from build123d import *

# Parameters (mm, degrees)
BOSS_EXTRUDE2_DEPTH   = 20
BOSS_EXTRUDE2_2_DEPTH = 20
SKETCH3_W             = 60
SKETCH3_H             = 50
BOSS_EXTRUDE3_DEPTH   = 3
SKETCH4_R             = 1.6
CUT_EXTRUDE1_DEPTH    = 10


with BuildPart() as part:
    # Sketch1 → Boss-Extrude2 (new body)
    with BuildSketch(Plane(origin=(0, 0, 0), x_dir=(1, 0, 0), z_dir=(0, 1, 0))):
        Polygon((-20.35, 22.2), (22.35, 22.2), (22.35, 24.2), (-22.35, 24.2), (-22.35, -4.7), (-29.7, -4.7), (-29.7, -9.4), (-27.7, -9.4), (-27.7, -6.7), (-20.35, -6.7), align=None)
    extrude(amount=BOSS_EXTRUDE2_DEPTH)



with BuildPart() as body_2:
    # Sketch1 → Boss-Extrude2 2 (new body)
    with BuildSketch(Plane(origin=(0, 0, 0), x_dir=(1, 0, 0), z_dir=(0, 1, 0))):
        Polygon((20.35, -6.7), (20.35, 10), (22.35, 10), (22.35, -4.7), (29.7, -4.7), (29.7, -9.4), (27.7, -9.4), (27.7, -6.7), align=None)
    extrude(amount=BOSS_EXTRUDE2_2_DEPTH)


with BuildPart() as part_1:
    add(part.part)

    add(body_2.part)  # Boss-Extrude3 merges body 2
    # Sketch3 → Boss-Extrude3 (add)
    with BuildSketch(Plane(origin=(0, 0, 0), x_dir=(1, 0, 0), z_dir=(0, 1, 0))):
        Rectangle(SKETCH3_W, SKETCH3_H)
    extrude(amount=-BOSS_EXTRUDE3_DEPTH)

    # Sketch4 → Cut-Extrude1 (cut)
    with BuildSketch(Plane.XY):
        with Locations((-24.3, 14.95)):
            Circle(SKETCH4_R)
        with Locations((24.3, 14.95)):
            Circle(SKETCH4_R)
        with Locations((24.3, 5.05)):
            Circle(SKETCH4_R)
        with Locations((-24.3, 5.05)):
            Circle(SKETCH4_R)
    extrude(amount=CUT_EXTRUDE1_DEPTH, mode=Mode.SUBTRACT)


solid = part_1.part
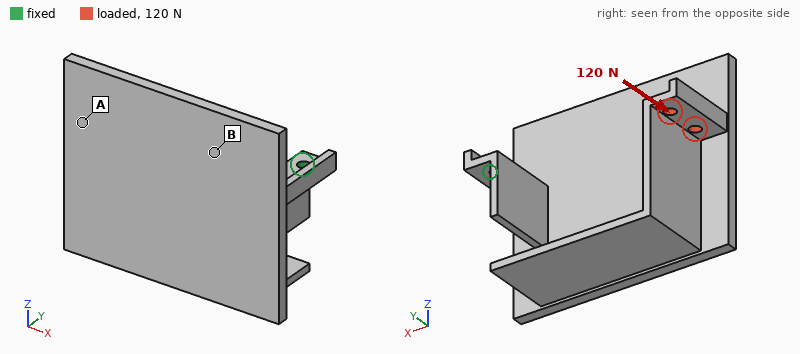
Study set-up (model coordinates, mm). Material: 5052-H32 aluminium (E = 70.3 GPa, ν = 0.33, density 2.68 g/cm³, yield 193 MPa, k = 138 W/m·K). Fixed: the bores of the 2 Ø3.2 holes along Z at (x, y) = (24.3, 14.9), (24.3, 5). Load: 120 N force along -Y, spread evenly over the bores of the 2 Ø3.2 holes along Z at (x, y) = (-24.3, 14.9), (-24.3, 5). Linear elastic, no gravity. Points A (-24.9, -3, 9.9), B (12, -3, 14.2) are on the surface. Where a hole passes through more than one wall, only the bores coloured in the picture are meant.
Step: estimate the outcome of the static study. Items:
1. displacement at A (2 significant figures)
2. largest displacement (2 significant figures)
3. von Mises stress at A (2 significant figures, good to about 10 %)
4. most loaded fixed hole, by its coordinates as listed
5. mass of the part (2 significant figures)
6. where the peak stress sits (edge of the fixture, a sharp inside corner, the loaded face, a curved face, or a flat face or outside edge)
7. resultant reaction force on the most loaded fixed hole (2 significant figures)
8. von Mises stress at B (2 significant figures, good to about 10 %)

0.74 mm
0.91 mm
17 MPa
(24.3, 5)
36 g
edge of the fixture
360 N
54 MPa
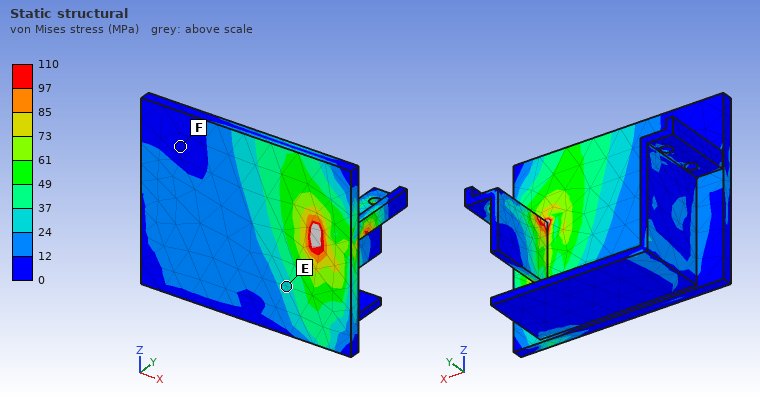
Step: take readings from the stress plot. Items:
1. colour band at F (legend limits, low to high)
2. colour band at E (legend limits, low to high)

0 to 12 MPa
24 to 37 MPa
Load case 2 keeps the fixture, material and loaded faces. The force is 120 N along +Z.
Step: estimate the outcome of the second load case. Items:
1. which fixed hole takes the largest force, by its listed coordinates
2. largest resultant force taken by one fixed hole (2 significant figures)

(24.3, 5)
110 N
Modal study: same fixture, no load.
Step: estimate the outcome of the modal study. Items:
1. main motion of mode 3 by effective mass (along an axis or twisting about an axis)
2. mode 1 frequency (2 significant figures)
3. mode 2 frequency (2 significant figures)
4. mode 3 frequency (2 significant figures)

twisting about X
540 Hz
550 Hz
1300 Hz
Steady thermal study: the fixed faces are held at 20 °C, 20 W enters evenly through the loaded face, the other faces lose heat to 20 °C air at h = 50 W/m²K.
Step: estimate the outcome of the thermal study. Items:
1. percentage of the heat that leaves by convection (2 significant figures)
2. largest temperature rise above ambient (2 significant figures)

63 %
69 K
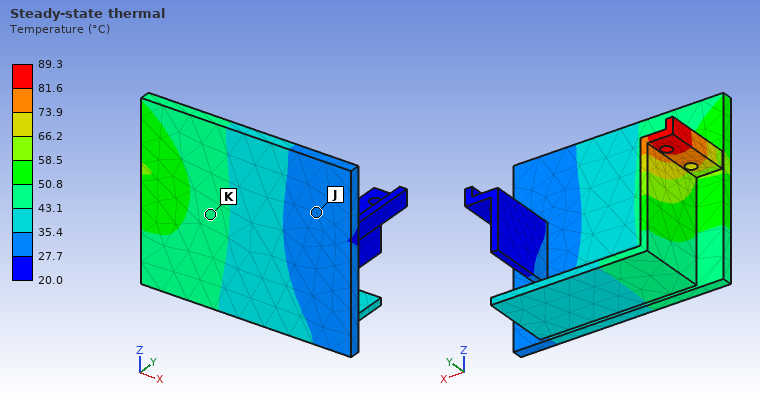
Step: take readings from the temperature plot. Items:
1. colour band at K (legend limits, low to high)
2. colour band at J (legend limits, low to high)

43.1 to 50.8 °C
27.7 to 35.4 °C
